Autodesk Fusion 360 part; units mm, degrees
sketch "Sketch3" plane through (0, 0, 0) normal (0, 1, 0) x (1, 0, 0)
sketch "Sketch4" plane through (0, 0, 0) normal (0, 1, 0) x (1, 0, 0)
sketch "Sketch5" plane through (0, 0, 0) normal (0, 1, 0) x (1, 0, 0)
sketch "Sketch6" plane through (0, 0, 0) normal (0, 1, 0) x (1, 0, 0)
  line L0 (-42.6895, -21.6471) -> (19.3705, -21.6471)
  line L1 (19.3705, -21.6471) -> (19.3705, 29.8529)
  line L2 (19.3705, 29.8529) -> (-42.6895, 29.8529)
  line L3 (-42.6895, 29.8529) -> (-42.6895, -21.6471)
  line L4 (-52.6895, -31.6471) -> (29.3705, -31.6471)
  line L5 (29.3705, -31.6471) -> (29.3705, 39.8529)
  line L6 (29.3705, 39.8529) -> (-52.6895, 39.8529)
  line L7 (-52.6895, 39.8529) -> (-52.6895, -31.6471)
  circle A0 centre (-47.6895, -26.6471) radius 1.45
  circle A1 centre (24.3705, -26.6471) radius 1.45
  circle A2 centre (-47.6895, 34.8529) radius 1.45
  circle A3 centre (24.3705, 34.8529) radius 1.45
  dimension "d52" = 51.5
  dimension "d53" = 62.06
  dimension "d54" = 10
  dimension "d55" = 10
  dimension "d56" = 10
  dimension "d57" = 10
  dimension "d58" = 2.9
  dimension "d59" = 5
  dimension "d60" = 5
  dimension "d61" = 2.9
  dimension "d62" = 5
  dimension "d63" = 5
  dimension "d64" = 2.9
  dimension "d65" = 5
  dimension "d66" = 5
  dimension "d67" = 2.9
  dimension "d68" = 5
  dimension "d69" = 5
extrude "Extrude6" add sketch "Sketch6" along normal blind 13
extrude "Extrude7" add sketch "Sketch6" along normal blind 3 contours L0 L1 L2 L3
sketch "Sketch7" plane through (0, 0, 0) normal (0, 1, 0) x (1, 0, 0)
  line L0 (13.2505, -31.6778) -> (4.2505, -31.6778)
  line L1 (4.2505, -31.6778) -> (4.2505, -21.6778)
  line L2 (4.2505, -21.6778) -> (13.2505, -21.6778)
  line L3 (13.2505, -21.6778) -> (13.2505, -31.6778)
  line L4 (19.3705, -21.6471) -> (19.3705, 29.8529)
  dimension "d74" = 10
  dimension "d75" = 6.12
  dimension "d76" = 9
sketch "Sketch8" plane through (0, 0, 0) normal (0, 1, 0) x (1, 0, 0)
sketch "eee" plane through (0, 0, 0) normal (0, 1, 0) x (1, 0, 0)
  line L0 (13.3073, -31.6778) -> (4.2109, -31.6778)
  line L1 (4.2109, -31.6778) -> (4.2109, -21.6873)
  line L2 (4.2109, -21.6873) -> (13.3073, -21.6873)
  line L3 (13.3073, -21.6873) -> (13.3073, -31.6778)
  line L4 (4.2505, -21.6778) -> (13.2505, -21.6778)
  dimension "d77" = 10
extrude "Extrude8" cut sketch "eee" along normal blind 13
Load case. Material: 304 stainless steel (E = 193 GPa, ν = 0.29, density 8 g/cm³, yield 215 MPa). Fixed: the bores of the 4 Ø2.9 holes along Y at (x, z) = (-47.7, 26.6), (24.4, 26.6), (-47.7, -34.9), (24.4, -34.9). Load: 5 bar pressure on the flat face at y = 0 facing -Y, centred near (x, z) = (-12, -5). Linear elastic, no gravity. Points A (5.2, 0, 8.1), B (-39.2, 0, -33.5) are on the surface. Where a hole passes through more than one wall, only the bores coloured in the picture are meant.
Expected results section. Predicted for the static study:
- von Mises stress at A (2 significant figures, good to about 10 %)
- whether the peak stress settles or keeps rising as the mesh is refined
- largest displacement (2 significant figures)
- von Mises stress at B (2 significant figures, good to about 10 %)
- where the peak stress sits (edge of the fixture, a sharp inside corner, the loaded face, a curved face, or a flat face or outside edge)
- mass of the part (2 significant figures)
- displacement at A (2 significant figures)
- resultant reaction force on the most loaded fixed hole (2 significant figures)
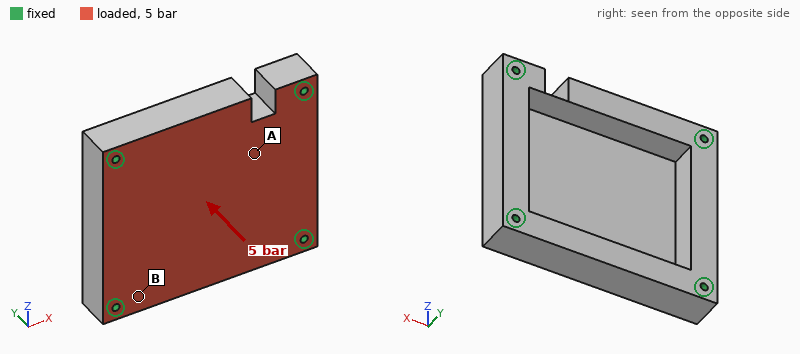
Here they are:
18 MPa
keeps rising
25 µm
9.6 MPa
a sharp inside corner
340 g
15 µm
930 N
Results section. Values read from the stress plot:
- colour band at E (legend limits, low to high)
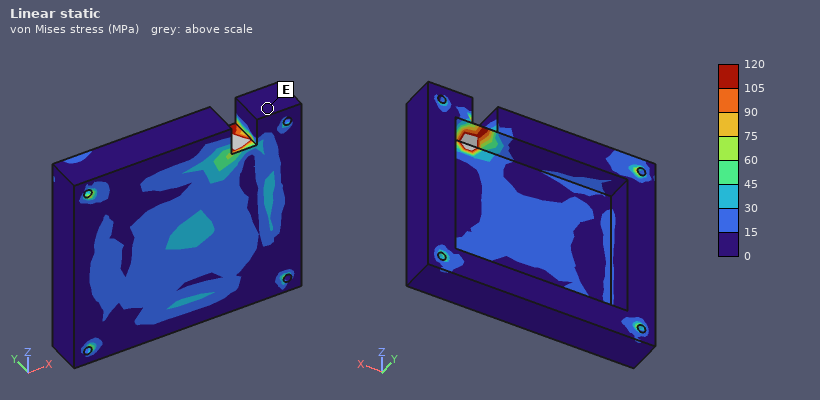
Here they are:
0 to 15 MPa
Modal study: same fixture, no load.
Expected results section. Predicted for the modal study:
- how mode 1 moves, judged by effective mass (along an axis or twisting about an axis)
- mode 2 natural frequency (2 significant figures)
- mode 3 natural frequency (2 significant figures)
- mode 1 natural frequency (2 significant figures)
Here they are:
along Y
6600 Hz
9700 Hz
5500 Hz
